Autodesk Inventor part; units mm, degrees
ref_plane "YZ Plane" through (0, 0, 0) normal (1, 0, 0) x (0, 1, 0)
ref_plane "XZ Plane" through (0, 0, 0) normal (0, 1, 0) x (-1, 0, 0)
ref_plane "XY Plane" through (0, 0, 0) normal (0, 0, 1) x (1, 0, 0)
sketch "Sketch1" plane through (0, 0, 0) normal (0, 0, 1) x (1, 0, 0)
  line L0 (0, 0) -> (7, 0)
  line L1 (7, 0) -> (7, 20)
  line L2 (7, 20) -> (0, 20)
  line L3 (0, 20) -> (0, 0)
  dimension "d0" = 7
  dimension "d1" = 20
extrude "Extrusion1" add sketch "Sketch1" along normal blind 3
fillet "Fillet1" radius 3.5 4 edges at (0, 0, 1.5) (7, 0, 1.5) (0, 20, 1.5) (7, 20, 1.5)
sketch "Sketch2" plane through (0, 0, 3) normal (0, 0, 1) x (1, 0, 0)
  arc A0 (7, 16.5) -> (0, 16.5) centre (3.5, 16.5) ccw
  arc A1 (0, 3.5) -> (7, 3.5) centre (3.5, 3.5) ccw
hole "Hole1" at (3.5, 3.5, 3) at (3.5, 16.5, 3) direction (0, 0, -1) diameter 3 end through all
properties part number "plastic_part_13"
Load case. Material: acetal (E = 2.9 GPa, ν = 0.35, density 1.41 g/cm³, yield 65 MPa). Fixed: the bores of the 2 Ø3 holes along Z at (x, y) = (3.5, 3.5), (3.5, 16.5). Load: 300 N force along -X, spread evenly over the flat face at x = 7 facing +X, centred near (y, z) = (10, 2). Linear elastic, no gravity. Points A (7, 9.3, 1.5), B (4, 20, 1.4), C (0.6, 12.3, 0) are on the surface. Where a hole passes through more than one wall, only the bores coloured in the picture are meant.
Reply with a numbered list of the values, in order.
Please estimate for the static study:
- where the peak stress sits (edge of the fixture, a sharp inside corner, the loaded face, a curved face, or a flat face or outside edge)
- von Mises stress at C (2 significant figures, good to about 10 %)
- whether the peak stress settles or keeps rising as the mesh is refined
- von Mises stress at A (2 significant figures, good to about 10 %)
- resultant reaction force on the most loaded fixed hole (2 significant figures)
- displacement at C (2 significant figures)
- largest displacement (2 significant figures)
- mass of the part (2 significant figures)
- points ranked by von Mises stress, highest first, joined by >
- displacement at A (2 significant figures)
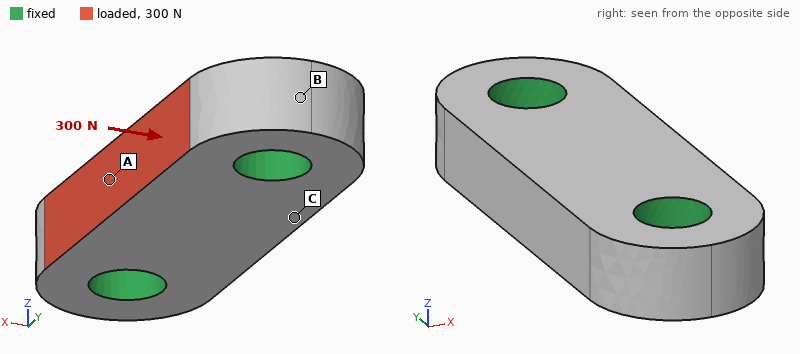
1. edge of the fixture
2. 5.2 MPa
3. keeps rising
4. 11 MPa
5. 150 N
6. 19 µm
7. 32 µm
8. 0.49 g
9. A > C > B
10. 31 µm
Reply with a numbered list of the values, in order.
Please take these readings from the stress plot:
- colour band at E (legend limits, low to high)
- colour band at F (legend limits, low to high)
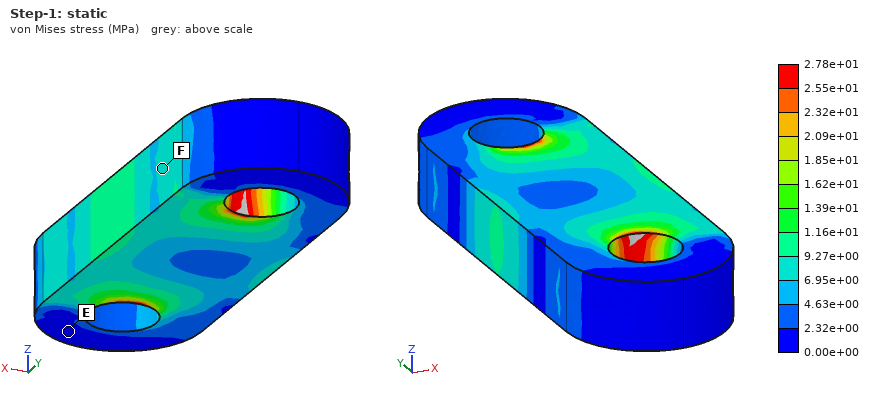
1. 0.00e+00 to 2.32e+00 MPa
2. 6.95e+00 to 9.27e+00 MPa
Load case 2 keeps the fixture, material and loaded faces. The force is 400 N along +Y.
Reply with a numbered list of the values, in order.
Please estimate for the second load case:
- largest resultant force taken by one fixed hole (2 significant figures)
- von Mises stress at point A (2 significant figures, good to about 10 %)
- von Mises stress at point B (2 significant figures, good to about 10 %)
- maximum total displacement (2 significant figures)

1. 220 N
2. 18 MPa
3. 3.3 MPa
4. 30 µm
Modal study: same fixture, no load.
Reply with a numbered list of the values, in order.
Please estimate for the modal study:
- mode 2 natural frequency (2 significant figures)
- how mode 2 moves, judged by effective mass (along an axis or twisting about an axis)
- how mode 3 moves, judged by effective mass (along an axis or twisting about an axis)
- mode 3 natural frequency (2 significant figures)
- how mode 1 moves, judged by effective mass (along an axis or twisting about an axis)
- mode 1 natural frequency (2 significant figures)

1. 28 kHz
2. twisting about Y
3. along X
4. 30 kHz
5. along Z
6. 24 kHz
